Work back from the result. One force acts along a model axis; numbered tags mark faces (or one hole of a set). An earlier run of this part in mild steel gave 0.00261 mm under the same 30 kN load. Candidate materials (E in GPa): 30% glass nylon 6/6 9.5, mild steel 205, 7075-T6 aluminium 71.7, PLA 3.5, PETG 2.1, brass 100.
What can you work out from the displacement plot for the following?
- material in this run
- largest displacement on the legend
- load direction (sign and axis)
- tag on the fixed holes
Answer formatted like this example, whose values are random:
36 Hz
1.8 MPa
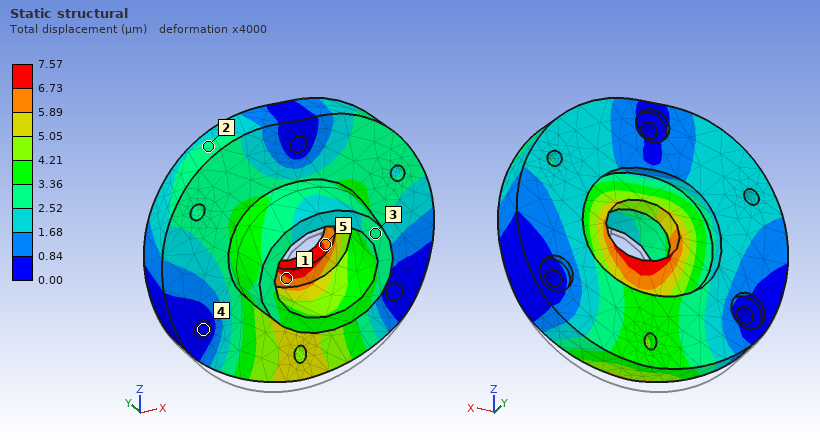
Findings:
7075-T6 aluminium
7.57 µm
+Z
4
